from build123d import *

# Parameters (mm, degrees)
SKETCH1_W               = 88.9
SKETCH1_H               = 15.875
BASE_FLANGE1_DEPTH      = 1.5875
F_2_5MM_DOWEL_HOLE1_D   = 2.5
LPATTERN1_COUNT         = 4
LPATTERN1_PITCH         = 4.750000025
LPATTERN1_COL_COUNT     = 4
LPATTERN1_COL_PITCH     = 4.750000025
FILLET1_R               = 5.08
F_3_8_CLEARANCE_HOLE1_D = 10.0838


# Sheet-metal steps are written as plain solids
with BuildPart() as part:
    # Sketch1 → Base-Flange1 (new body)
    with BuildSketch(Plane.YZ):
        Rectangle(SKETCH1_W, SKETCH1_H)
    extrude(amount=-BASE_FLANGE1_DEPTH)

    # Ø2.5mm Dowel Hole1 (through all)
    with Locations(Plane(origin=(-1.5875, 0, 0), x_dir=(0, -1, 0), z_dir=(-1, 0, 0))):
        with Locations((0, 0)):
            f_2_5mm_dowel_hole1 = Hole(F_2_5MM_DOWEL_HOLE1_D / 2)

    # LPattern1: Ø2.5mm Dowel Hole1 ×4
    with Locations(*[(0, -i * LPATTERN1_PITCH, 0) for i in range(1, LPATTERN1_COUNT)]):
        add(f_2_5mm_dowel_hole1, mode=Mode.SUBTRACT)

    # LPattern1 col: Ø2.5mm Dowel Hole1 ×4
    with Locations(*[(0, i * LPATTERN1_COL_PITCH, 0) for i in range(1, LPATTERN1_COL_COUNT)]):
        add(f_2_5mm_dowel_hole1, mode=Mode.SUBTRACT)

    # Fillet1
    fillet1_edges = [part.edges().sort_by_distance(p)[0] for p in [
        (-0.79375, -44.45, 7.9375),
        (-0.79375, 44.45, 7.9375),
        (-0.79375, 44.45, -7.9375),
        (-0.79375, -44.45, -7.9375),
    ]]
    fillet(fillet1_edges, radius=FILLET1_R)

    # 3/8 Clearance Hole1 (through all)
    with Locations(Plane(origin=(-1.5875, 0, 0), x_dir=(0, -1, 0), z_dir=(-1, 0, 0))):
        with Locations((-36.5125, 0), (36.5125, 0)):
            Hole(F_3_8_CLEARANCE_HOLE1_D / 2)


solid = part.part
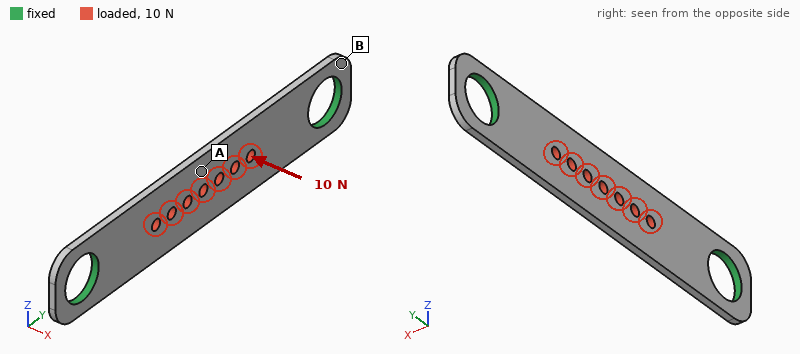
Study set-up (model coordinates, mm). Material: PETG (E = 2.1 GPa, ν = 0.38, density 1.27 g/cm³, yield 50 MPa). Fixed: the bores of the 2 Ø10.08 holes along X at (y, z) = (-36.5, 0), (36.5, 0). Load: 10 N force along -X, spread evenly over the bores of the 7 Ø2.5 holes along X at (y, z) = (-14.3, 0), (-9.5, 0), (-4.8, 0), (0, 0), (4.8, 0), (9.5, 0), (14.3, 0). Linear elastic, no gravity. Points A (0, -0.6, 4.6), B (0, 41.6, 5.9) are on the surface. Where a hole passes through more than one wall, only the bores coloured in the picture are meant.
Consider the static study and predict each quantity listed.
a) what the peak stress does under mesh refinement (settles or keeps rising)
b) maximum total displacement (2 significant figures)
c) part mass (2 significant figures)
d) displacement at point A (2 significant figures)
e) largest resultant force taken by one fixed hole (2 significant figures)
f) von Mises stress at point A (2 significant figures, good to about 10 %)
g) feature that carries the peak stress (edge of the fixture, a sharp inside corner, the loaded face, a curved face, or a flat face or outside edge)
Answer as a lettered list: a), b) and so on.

a) keeps rising
b) 1.0 mm
c) 2.4 g
d) 1.00 mm
e) 5.0 N
f) 7.0 MPa
g) edge of the fixture
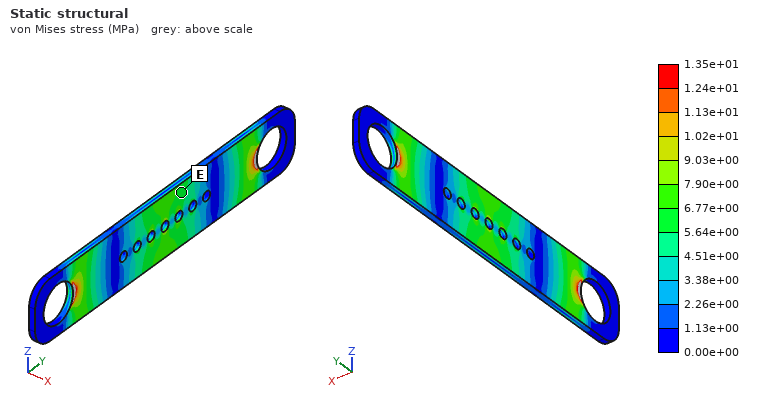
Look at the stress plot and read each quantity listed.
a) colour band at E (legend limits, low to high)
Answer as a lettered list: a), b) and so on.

a) 5.64e+00 to 6.77e+00 MPa
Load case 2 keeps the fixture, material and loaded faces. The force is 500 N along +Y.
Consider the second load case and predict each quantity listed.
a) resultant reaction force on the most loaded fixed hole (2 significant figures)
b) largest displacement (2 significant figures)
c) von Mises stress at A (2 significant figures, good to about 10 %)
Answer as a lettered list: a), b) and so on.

a) 250 N
b) 0.15 mm
c) 4.1 MPa
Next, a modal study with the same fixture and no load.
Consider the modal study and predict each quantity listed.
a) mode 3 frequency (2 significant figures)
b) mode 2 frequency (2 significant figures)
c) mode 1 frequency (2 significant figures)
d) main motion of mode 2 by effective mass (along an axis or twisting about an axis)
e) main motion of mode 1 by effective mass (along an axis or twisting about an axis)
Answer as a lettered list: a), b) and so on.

a) 1400 Hz
b) 1300 Hz
c) 520 Hz
d) twisting about Y
e) along X
